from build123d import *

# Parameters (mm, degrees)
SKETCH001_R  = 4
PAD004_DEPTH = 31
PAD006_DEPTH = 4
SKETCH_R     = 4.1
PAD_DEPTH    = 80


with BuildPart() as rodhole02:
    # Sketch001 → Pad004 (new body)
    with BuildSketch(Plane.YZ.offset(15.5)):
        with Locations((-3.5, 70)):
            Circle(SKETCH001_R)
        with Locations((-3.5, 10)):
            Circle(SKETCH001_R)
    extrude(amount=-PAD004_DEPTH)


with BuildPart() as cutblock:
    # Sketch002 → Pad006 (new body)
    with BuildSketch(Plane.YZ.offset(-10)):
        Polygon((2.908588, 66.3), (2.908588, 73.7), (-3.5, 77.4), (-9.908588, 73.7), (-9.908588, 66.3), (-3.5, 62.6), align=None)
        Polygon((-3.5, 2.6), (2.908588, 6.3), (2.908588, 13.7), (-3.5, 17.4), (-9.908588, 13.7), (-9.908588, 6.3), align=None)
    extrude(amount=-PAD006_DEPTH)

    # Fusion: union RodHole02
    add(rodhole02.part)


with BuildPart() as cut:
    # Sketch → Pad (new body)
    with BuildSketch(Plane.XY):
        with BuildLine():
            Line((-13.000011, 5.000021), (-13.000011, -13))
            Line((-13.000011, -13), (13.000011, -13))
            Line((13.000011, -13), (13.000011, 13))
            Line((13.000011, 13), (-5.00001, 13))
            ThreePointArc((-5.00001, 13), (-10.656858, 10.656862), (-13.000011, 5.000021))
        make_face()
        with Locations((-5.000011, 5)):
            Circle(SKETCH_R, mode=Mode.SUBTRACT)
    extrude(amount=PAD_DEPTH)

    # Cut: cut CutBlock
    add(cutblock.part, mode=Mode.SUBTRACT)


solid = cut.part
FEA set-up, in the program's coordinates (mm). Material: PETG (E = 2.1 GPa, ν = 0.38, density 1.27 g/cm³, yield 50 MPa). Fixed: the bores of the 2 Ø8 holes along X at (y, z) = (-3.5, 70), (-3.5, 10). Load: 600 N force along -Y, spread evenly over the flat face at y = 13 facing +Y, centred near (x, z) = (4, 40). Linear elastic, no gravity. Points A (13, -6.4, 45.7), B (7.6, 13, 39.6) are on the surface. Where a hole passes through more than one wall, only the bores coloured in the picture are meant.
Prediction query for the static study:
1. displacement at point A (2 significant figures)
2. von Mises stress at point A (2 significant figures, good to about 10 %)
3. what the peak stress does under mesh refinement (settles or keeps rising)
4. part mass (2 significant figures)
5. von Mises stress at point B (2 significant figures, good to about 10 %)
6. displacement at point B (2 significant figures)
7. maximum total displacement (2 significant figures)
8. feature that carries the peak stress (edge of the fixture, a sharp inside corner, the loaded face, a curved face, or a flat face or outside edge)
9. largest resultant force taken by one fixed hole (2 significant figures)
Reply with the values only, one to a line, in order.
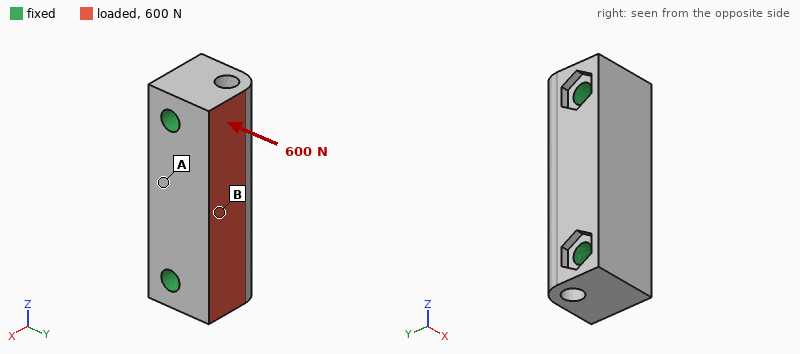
16 µm
0.26 MPa
keeps rising
58 g
0.80 MPa
17 µm
18 µm
edge of the fixture
310 N
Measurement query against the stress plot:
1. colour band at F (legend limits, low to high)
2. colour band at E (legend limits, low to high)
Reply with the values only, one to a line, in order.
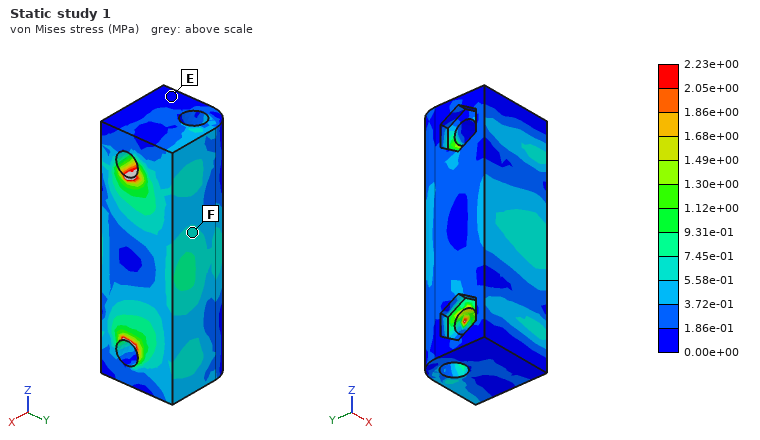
5.58e-01 to 7.45e-01 MPa
0.00e+00 to 1.86e-01 MPa
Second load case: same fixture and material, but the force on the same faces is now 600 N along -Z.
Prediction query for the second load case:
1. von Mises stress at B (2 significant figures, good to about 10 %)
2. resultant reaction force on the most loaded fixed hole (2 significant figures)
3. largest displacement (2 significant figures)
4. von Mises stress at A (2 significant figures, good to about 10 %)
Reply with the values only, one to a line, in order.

0.72 MPa
330 N
19 µm
0.34 MPa
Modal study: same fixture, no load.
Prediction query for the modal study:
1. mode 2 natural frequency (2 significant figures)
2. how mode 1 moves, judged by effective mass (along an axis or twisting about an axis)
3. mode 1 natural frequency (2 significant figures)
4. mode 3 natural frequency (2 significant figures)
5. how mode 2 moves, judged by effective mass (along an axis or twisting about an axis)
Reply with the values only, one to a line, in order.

4600 Hz
along Y
4300 Hz
5600 Hz
along X
